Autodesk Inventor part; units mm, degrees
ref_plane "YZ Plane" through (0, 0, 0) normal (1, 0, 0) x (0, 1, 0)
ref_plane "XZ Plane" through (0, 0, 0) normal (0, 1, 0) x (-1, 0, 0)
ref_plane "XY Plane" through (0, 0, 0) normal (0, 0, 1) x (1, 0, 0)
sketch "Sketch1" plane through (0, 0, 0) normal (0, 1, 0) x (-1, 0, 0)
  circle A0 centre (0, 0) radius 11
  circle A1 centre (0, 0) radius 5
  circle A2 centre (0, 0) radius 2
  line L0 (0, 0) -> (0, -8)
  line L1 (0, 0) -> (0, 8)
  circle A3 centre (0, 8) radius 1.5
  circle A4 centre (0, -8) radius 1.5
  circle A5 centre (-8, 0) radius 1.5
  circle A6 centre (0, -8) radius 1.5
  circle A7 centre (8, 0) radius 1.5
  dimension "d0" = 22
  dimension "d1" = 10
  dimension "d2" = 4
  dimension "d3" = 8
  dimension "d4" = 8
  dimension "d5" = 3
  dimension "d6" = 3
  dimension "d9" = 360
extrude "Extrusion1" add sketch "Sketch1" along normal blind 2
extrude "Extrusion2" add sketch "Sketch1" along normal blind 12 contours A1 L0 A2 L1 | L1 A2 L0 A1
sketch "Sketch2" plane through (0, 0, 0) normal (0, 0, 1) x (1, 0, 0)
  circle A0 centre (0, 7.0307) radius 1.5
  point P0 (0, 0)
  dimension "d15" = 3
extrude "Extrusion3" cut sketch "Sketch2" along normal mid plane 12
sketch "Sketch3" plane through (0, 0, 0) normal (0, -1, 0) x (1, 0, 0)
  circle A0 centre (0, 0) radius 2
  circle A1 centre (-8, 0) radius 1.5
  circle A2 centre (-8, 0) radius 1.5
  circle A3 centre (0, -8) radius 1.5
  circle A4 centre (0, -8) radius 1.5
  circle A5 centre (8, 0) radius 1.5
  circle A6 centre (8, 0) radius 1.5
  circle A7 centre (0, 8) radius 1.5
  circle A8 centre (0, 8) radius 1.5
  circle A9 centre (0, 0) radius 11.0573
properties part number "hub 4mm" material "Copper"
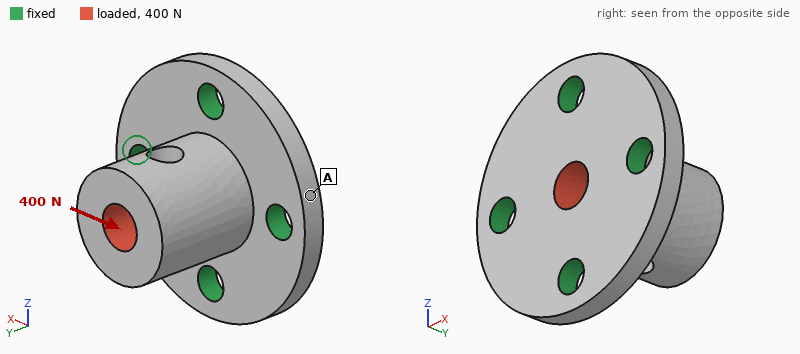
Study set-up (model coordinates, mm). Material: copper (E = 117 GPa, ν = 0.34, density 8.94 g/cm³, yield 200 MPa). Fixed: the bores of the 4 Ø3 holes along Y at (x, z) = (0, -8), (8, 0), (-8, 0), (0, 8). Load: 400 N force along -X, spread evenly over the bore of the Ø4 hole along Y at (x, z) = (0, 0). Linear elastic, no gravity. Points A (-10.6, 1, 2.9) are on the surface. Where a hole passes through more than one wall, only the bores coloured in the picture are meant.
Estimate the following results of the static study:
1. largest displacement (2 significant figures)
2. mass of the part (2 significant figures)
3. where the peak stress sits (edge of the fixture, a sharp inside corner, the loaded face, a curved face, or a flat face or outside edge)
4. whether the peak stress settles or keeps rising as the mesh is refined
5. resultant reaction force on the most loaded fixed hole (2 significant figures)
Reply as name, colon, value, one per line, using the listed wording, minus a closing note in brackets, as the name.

largest displacement: 5.0 µm
mass of the part: 12 g
where the peak stress sits: edge of the fixture
whether the peak stress settles or keeps rising as the mesh is refined: keeps rising
resultant reaction force on the most loaded fixed hole: 200 N
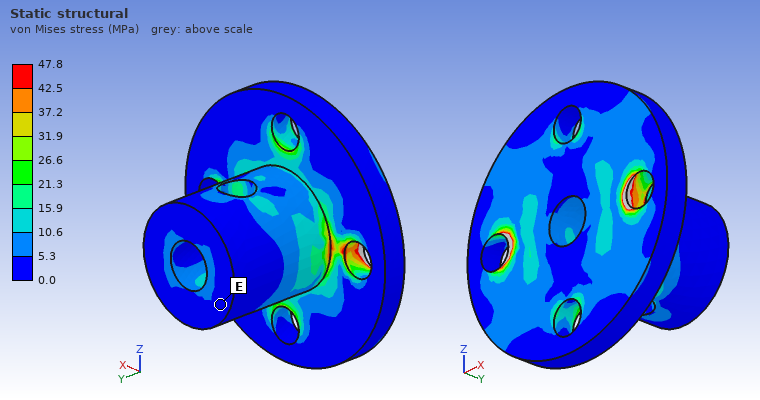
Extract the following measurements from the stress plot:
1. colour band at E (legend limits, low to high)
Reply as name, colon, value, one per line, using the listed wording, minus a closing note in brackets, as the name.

colour band at E: 0.0 to 5.3 MPa
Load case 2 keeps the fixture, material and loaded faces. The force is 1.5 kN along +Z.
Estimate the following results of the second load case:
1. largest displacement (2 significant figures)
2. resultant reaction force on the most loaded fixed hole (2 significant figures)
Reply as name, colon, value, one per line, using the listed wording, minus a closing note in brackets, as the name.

largest displacement: 18 µm
resultant reaction force on the most loaded fixed hole: 760 N
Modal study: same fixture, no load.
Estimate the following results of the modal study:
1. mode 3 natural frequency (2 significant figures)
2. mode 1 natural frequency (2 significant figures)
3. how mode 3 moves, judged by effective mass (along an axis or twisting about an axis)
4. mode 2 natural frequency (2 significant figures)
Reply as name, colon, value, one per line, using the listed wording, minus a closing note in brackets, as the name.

mode 3 natural frequency: 35 kHz
mode 1 natural frequency: 20 kHz
how mode 3 moves, judged by effective mass: along Y
mode 2 natural frequency: 21 kHz
